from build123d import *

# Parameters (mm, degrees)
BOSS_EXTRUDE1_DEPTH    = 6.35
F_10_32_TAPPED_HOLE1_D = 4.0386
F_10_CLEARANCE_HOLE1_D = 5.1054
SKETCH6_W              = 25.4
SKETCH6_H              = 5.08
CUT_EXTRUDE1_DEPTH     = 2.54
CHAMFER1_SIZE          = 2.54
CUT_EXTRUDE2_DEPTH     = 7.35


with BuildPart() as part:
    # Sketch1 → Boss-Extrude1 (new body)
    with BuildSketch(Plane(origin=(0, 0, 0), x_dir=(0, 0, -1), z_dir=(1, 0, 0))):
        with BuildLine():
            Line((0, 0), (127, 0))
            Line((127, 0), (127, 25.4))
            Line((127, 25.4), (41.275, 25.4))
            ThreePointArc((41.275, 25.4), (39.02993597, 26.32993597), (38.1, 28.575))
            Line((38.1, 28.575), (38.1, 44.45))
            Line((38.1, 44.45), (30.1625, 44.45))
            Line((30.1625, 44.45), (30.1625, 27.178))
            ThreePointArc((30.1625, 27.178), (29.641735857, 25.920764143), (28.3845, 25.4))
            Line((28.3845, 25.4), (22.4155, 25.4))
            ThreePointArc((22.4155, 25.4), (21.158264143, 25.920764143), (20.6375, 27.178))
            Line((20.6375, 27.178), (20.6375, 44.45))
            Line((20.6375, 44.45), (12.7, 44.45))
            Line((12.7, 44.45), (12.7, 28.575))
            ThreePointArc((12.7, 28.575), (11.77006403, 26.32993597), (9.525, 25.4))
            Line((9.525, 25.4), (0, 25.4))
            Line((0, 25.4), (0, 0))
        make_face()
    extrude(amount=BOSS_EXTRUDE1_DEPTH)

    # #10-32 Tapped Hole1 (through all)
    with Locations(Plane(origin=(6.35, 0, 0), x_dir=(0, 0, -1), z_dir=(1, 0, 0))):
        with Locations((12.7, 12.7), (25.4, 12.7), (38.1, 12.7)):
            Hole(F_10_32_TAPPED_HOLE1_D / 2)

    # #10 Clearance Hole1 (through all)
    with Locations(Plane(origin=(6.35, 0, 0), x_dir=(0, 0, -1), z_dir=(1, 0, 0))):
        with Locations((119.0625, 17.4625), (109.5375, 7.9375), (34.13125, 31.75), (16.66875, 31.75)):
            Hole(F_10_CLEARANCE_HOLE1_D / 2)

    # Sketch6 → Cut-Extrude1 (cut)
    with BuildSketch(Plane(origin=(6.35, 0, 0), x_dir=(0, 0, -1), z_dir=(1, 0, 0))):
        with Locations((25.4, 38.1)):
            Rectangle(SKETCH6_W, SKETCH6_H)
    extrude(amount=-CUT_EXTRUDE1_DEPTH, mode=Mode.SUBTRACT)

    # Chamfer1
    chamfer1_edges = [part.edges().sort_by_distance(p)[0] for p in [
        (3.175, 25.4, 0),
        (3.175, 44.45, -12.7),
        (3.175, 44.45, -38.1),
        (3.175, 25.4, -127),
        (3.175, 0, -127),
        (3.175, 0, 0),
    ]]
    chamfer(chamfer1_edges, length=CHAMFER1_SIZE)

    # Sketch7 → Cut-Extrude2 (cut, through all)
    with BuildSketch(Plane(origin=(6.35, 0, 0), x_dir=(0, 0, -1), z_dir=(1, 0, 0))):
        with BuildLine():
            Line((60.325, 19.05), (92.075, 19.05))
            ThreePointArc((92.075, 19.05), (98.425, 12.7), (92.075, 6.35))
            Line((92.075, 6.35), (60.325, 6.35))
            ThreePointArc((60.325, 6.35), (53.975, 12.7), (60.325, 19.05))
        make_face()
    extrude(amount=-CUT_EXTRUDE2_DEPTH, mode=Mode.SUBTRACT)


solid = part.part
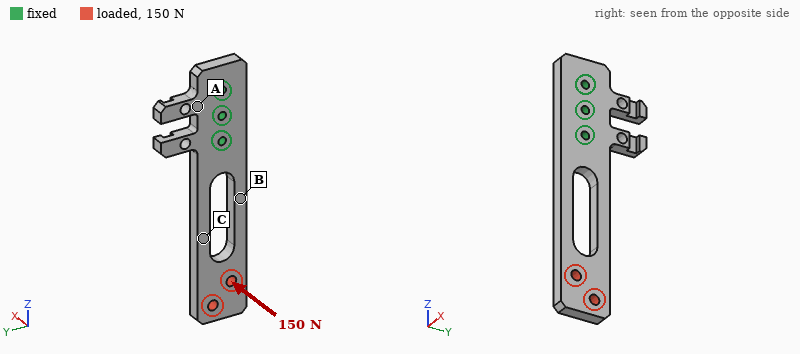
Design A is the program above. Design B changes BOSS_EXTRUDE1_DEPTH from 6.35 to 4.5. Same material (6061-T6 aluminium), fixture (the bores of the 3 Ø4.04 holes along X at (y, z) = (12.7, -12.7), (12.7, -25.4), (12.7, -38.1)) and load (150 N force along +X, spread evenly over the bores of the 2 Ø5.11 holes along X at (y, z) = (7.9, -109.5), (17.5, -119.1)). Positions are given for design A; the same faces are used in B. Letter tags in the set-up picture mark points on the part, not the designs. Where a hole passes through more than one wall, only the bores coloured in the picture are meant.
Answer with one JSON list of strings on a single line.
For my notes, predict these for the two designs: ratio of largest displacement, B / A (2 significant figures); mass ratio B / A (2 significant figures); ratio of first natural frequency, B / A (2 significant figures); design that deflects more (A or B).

["2.8", "0.71", "0.72", "B"]
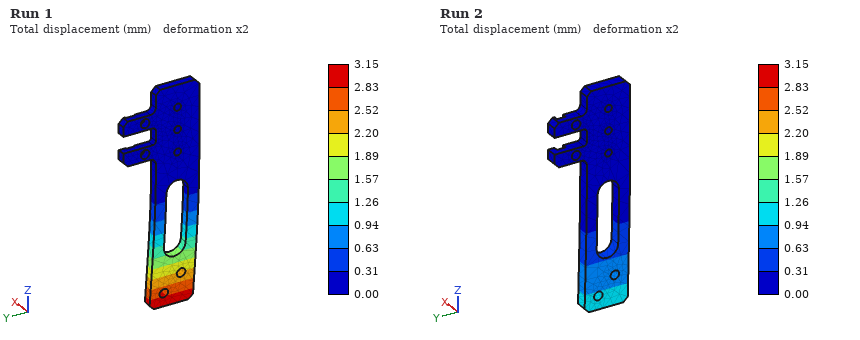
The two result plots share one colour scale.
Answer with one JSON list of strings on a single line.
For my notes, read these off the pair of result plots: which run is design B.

["Run 1"]
